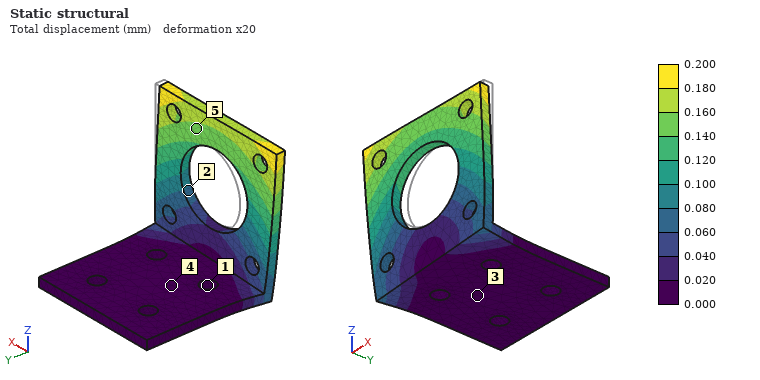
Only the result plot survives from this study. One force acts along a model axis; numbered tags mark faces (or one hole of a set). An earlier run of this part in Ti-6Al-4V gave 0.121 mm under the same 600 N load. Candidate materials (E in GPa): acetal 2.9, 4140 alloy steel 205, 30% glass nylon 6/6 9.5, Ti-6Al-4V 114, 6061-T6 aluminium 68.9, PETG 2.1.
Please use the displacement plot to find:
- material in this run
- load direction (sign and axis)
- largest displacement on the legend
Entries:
6061-T6 aluminium
-X
0.200 mm
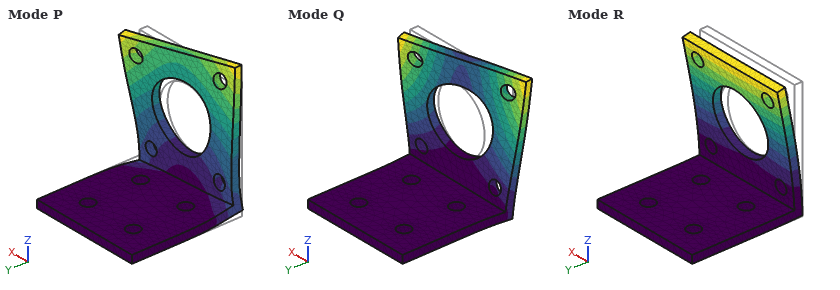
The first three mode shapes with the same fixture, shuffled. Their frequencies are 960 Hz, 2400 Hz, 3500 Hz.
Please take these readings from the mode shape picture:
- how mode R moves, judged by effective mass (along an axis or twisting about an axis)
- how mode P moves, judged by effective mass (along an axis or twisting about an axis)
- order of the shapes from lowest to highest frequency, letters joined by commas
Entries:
along Y
along X
R, Q, P
